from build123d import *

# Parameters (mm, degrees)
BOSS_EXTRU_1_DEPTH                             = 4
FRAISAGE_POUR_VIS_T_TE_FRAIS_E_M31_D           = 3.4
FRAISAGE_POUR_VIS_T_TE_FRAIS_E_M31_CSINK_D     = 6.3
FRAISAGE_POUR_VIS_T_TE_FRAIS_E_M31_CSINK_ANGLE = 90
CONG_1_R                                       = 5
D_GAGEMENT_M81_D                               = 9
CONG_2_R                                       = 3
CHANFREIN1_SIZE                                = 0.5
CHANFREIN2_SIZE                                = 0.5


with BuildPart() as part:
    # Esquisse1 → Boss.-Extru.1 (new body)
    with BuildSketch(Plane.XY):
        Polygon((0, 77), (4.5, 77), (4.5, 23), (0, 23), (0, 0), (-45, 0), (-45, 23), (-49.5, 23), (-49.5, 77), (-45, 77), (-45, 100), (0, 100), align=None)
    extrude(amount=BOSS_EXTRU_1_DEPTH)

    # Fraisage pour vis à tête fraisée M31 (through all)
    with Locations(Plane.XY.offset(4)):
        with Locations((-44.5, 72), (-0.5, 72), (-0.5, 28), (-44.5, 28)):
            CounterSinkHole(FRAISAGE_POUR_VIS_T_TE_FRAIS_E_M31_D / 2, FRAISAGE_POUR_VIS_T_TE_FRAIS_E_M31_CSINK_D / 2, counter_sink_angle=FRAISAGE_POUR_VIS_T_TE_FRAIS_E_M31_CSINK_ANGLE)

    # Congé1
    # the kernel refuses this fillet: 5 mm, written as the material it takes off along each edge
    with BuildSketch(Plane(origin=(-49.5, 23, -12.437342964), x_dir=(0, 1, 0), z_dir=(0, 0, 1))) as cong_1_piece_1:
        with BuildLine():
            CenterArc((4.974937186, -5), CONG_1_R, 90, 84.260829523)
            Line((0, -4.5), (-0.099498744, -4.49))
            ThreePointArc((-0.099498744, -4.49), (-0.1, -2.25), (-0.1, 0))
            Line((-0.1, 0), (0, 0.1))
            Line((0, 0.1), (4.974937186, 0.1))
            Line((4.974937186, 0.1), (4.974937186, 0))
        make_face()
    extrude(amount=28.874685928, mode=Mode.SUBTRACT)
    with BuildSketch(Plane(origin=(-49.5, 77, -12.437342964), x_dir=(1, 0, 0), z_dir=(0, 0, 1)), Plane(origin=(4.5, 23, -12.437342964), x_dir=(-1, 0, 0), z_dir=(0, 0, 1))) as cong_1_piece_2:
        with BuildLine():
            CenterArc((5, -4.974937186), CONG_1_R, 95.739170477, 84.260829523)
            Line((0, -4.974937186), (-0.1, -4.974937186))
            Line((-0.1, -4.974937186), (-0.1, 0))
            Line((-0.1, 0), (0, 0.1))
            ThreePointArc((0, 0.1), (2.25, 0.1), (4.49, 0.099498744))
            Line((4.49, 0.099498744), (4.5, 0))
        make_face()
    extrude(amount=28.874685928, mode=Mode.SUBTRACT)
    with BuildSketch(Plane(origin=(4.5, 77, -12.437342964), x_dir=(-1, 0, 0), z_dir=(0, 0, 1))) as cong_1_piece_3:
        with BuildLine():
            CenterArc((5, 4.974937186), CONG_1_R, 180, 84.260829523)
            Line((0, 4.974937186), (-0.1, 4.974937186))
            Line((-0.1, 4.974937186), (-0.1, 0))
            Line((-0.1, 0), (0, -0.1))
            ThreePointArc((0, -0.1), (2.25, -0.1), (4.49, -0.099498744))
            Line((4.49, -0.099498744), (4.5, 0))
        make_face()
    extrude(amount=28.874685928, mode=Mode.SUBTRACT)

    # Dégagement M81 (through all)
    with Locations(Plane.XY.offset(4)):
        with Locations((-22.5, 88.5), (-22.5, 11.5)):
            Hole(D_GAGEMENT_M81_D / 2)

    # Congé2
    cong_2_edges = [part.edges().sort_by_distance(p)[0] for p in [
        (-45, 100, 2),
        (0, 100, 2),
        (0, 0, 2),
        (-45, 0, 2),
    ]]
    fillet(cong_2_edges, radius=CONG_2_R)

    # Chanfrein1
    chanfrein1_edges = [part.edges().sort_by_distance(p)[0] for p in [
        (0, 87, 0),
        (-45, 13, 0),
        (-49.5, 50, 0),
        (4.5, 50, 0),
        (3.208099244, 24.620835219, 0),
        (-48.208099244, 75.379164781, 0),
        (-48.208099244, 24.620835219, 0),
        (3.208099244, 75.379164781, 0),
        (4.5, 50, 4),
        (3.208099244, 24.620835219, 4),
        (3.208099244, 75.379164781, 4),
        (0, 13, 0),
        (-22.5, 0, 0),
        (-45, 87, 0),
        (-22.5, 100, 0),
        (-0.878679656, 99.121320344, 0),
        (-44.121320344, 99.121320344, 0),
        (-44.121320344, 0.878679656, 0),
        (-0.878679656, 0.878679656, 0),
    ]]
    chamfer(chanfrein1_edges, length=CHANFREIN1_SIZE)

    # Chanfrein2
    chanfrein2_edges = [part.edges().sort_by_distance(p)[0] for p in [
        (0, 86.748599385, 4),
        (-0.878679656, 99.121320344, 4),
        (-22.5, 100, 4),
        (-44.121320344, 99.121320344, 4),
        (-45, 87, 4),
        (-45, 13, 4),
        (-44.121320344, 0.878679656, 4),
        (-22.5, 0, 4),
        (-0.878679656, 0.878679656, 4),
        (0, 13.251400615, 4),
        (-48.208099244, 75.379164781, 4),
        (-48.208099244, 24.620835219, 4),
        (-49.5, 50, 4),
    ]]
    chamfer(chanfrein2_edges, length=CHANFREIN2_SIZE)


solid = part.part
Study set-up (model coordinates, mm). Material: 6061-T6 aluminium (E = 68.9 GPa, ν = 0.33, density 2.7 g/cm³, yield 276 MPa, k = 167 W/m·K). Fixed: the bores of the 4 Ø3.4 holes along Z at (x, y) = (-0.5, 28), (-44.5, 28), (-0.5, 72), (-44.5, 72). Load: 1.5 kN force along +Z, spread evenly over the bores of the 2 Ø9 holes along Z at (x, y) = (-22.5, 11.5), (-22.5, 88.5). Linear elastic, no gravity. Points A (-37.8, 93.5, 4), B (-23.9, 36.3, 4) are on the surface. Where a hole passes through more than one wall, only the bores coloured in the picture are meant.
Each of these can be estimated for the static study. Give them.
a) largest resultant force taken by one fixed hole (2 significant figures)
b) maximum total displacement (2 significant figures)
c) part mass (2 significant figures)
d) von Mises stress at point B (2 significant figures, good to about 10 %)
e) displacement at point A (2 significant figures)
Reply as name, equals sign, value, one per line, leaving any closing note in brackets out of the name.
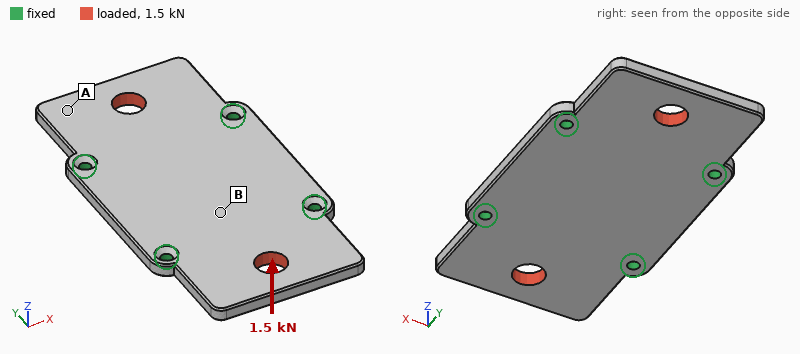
largest resultant force taken by one fixed hole = 540 N
maximum total displacement = 0.34 mm
part mass = 51 g
von Mises stress at point B = 48 MPa
displacement at point A = 0.21 mm
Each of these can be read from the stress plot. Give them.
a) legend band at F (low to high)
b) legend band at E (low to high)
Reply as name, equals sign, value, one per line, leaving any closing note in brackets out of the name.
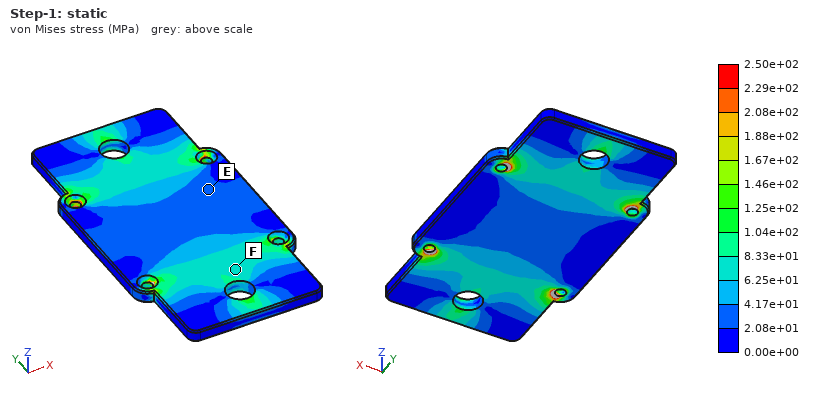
legend band at F = 6.25e+01 to 8.33e+01 MPa
legend band at E = 2.08e+01 to 4.17e+01 MPa
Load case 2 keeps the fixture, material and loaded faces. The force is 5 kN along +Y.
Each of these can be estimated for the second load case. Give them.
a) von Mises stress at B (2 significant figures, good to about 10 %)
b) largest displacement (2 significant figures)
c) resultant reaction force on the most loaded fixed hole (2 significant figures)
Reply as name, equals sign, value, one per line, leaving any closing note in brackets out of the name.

von Mises stress at B = 10 MPa
largest displacement = 16 µm
resultant reaction force on the most loaded fixed hole = 1.3 kN
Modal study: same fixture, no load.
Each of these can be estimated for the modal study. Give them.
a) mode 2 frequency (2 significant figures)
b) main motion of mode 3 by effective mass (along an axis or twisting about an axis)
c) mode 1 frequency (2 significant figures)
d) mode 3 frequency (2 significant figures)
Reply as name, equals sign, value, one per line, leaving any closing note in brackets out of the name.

mode 2 frequency = 3100 Hz
main motion of mode 3 by effective mass = along Z
mode 1 frequency = 3000 Hz
mode 3 frequency = 6500 Hz
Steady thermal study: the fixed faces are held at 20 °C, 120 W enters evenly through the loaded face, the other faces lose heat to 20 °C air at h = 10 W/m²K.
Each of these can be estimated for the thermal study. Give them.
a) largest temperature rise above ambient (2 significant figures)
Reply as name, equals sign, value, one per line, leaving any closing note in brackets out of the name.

largest temperature rise above ambient = 69 K
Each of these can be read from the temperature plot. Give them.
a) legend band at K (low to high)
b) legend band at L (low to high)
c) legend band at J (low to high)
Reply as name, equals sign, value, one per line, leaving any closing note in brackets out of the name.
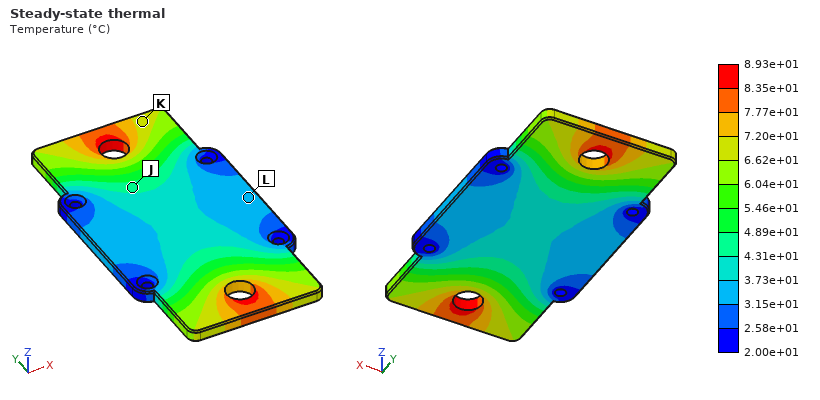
legend band at K = 6.62e+01 to 7.20e+01 °C
legend band at L = 3.15e+01 to 3.73e+01 °C
legend band at J = 4.31e+01 to 4.89e+01 °C
